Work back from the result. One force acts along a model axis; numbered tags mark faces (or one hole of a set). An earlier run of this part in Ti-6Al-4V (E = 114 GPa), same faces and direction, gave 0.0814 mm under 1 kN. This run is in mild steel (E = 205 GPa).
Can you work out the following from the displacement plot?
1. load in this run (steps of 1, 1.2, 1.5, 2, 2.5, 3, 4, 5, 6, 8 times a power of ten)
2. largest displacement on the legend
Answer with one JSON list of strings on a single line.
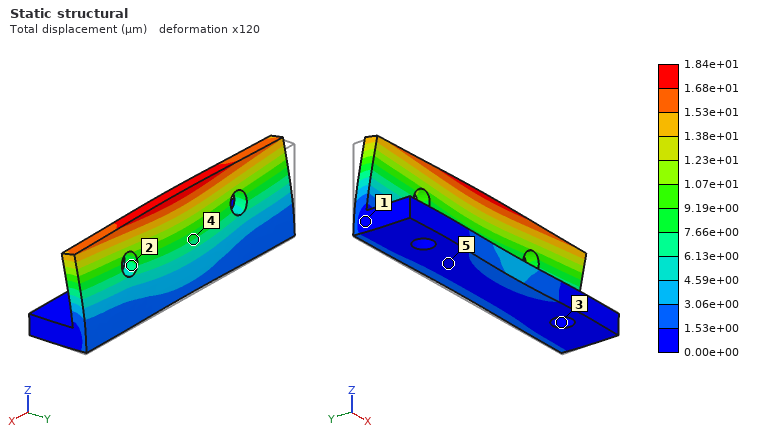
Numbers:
["400 N", "1.84e+01 µm"]
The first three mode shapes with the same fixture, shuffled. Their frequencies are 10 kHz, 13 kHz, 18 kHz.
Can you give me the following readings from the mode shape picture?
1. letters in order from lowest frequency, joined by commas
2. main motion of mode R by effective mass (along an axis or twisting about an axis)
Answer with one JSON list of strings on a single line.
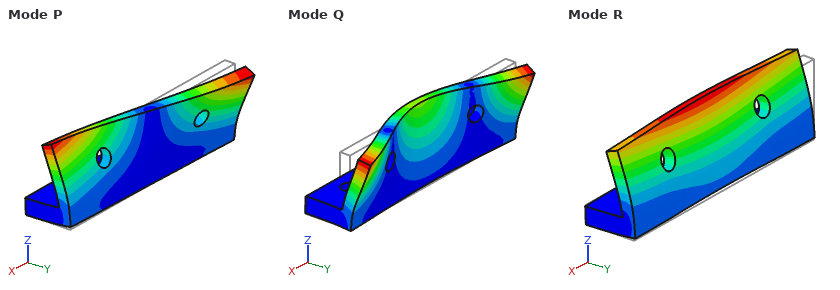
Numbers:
["R, P, Q", "along Y"]
